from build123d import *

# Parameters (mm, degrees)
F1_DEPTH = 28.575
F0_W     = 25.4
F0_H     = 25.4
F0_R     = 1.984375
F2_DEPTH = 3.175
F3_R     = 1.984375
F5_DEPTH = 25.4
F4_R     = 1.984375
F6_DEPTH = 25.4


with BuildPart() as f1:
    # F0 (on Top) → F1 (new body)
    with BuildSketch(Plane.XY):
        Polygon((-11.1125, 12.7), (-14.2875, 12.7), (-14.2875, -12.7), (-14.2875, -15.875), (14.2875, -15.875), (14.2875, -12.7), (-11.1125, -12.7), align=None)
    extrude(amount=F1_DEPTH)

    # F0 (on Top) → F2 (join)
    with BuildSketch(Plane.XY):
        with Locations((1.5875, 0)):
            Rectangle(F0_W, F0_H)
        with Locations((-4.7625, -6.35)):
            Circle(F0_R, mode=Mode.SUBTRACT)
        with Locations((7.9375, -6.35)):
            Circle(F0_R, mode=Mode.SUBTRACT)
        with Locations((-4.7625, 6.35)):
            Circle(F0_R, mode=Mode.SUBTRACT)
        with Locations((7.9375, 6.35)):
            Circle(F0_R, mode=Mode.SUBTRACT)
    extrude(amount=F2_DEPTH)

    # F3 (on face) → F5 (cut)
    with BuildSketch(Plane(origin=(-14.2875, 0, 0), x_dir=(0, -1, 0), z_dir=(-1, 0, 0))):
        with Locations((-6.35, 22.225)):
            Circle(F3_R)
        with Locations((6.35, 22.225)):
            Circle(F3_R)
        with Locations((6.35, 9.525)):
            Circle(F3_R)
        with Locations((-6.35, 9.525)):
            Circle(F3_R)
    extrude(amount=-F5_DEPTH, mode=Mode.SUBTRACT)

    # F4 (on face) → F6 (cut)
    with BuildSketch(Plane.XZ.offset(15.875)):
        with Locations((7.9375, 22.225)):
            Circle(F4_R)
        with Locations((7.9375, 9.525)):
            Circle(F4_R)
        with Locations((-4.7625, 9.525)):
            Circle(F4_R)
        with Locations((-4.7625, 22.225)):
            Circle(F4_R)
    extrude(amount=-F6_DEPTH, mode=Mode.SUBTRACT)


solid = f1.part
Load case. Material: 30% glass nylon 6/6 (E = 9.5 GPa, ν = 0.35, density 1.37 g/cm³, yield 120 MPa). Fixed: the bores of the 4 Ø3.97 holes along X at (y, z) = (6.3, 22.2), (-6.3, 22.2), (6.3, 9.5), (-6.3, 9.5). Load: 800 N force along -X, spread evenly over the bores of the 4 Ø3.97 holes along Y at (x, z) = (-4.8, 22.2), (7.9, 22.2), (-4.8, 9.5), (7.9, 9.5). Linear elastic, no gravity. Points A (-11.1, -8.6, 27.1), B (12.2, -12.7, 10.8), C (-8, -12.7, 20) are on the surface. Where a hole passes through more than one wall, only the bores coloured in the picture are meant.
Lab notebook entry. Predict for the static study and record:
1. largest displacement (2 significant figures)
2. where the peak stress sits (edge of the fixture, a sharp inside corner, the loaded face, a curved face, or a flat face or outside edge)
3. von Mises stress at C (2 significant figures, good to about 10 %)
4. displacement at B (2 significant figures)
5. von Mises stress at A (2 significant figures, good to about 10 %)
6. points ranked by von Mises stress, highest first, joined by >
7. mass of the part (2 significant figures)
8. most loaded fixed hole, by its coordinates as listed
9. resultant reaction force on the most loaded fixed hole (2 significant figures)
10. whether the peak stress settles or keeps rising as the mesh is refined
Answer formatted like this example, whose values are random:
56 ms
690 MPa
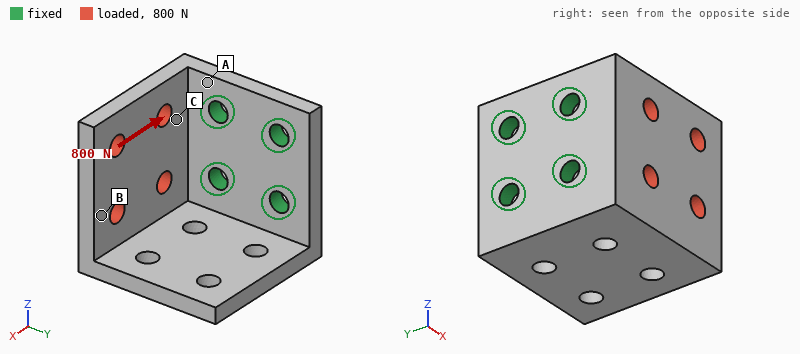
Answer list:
0.42 mm
edge of the fixture
30 MPa
0.24 mm
47 MPa
A > C > B
8.9 g
(-6.3, 9.5)
530 N
keeps rising
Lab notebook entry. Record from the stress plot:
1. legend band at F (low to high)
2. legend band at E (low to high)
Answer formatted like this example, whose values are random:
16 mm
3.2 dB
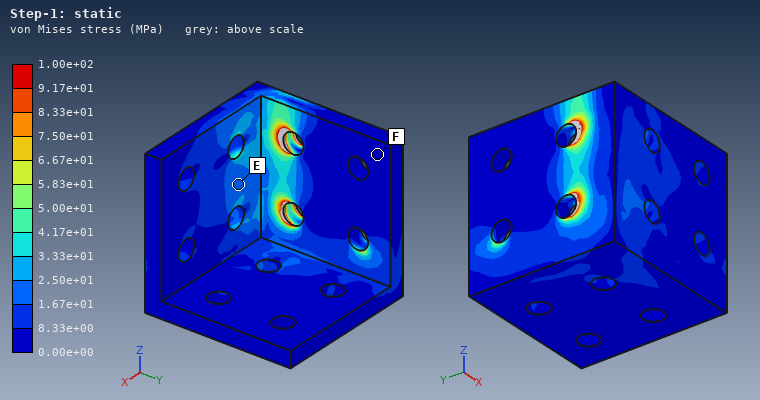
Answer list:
0.00e+00 to 8.33e+00 MPa
1.67e+01 to 2.50e+01 MPa
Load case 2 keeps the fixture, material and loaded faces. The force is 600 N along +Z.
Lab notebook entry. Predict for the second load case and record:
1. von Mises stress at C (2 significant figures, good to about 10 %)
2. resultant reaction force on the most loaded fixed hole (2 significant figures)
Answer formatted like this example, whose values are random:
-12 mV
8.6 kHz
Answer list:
48 MPa
650 N
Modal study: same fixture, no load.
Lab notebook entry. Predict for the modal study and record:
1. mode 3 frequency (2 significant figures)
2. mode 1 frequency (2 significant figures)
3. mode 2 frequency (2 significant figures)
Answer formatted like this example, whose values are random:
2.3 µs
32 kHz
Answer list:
3800 Hz
2100 Hz
2600 Hz
